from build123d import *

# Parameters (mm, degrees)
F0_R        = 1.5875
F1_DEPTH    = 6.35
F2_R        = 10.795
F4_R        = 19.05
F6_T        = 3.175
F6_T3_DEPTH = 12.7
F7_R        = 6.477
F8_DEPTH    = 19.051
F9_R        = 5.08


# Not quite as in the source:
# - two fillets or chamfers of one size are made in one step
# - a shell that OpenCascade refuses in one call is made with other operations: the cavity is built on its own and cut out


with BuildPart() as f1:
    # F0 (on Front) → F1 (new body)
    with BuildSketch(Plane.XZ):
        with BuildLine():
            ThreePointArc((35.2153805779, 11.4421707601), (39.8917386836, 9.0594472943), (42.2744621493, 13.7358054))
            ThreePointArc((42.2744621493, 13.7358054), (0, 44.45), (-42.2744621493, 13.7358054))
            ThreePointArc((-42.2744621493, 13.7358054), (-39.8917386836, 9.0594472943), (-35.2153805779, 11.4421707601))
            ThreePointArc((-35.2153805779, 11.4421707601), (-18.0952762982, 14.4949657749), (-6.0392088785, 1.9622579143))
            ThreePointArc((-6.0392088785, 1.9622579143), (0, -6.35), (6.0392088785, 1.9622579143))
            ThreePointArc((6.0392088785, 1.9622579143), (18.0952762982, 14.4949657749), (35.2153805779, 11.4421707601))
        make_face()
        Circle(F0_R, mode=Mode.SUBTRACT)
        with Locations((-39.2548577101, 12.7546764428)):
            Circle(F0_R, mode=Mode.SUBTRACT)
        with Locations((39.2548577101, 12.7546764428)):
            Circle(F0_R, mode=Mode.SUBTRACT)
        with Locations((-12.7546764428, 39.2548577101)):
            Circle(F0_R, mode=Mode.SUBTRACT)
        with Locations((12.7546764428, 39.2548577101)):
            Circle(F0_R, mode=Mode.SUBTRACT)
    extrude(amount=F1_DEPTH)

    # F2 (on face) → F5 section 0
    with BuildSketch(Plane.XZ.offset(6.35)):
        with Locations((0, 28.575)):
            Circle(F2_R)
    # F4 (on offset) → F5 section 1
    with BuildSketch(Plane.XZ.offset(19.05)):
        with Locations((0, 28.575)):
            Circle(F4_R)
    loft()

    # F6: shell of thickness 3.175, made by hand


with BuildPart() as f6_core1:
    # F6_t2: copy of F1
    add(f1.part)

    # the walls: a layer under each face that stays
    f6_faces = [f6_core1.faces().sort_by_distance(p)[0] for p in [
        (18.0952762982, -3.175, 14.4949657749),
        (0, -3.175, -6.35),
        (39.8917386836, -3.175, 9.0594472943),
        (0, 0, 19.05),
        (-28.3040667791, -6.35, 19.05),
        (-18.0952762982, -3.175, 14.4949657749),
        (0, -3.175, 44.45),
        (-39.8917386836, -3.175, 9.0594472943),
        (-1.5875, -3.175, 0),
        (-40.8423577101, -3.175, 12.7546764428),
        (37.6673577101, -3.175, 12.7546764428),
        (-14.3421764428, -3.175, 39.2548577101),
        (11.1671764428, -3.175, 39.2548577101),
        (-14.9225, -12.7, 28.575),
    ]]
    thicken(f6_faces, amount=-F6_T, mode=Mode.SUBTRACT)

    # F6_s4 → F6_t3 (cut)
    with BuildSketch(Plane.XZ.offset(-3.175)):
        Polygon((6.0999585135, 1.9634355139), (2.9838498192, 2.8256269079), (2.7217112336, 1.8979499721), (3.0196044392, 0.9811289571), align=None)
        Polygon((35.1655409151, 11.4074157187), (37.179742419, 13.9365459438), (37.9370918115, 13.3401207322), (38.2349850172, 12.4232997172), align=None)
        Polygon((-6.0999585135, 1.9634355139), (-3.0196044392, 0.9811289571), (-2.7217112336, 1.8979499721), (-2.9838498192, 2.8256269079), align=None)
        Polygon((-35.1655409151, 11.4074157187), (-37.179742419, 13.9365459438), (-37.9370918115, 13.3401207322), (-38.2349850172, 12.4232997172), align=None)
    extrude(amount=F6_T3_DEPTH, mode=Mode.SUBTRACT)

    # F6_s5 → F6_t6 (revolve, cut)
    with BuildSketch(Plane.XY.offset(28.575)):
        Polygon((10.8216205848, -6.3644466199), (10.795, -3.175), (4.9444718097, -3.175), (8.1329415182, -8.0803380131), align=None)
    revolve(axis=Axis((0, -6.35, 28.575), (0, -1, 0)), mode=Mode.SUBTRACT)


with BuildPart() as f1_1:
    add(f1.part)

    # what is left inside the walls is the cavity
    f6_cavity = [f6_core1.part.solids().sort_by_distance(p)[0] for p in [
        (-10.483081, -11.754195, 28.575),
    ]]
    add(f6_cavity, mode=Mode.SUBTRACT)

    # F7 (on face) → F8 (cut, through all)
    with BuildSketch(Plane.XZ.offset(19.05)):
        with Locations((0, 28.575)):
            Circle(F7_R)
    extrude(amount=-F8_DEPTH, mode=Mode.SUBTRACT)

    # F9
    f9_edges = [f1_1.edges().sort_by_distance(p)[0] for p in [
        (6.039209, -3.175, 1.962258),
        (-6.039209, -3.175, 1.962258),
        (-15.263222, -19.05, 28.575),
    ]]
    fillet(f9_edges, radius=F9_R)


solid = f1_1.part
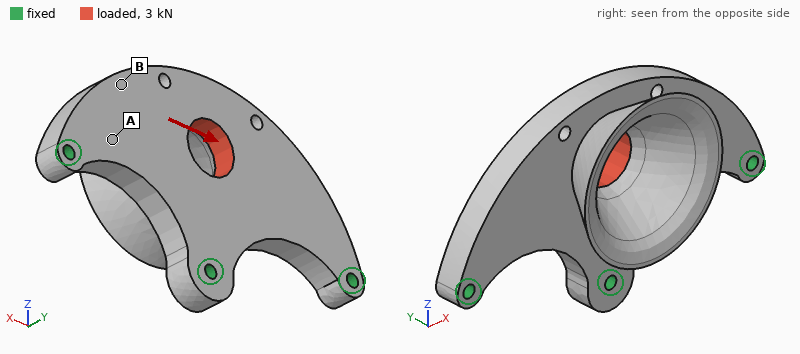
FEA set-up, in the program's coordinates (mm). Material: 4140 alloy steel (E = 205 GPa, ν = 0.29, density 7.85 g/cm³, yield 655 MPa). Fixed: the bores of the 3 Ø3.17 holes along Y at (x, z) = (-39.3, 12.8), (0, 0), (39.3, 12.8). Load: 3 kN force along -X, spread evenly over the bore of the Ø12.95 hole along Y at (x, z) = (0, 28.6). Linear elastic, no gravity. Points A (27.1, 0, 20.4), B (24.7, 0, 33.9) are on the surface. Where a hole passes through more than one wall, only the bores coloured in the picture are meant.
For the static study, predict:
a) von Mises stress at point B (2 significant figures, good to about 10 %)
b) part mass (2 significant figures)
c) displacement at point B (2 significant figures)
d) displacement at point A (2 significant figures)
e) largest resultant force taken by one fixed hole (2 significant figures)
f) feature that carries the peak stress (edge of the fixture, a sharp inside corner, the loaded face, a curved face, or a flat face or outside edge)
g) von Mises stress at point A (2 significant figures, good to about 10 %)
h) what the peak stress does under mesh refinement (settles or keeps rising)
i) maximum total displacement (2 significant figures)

7.3 MPa
130 g
2.9 µm
2.0 µm
1.3 kN
edge of the fixture
16 MPa
keeps rising
4.1 µm
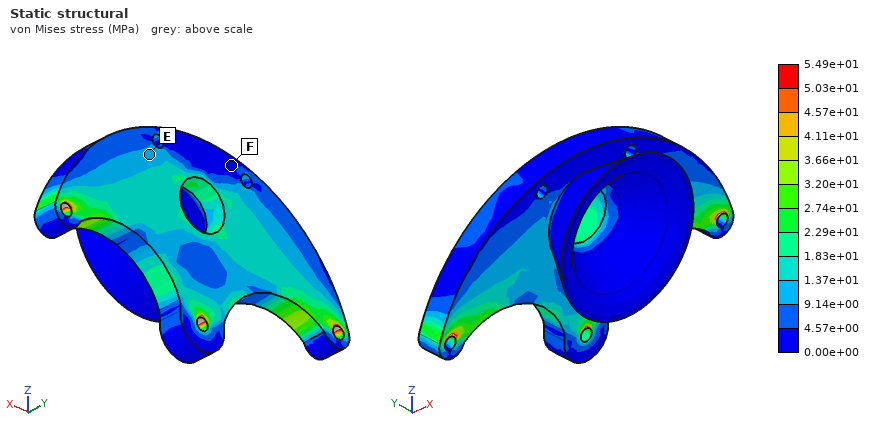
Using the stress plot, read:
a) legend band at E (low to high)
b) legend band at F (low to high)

9.14e+00 to 1.37e+01 MPa
0.00e+00 to 4.57e+00 MPa
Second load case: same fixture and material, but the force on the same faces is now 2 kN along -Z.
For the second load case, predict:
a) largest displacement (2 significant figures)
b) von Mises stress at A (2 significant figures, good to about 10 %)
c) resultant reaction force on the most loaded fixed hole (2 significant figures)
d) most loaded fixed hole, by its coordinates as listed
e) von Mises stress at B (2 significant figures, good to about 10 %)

4.2 µm
7.4 MPa
1.4 kN
(0, 0)
3.8 MPa
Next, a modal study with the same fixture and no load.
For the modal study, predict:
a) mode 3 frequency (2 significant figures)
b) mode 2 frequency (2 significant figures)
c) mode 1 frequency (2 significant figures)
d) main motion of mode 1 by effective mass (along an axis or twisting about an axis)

9600 Hz
6700 Hz
2500 Hz
along Y
